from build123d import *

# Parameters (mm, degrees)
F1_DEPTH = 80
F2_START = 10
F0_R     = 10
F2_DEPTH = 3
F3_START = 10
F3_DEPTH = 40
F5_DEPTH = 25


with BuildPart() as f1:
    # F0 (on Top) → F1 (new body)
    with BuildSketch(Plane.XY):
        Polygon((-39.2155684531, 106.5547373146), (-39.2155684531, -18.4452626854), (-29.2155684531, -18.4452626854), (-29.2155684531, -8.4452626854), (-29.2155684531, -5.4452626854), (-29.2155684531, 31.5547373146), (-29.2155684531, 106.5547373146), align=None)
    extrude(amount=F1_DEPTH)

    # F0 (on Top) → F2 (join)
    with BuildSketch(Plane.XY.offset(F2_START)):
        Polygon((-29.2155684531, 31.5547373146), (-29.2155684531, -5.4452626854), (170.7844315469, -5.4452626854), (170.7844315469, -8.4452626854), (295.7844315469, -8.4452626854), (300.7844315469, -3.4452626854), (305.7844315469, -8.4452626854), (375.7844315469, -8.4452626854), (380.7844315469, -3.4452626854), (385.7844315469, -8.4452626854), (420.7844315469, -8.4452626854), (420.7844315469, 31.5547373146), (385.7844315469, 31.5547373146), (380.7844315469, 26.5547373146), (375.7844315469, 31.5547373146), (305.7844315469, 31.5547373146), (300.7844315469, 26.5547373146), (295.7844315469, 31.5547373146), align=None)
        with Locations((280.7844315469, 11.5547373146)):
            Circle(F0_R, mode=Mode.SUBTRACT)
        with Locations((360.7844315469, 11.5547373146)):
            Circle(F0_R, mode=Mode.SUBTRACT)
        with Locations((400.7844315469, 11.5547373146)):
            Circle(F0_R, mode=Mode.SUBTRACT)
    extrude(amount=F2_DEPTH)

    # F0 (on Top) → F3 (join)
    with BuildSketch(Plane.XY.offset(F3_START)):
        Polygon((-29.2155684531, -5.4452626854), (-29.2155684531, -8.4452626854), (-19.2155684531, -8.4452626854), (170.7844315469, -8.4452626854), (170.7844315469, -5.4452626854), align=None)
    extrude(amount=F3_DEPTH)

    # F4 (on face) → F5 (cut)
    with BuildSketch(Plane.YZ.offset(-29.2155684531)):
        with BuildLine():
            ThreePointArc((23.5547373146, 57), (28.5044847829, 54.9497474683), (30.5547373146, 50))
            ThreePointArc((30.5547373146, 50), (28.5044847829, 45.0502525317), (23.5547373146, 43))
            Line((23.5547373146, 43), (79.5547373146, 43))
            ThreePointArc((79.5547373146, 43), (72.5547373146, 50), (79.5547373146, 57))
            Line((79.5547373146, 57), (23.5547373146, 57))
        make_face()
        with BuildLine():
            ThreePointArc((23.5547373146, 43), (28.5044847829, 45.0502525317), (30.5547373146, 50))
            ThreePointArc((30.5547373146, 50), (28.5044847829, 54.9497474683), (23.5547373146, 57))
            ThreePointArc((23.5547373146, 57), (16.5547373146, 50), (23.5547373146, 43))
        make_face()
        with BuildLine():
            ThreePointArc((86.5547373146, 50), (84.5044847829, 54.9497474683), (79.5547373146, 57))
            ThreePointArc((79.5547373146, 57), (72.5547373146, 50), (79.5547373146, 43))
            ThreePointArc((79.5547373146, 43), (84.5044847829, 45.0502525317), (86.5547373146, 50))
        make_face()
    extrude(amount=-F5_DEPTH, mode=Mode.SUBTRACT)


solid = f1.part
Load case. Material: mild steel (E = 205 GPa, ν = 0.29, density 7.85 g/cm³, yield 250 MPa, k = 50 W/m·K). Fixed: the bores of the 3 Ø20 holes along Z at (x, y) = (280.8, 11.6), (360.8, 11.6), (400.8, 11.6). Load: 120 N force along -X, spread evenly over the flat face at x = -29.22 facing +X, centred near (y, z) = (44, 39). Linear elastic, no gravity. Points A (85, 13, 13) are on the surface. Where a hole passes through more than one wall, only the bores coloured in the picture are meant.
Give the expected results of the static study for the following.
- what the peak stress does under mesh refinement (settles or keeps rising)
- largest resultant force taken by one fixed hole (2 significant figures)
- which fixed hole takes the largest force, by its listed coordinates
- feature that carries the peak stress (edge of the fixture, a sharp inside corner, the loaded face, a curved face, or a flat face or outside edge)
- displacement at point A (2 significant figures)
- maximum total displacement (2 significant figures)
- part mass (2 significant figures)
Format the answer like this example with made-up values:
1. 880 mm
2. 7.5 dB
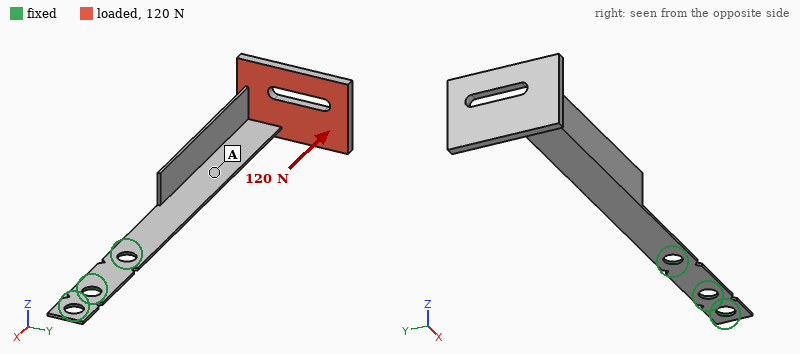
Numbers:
1. keeps rising
2. 120 N
3. (280.8, 11.6)
4. a sharp inside corner
5. 2.6 mm
6. 5.4 mm
7. 1.3 kg
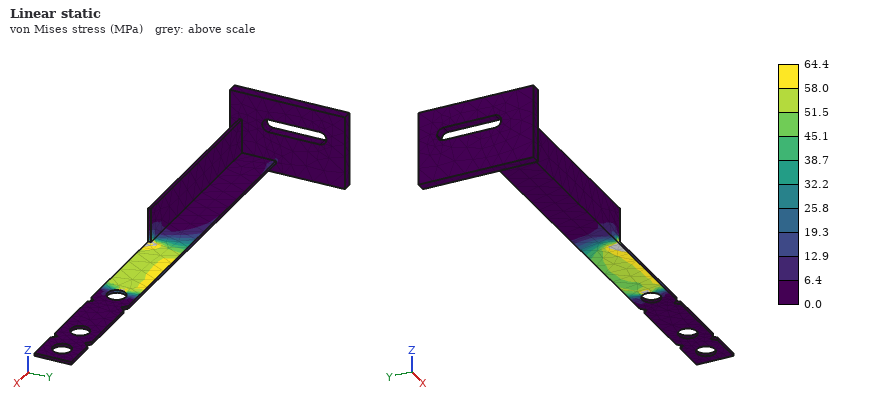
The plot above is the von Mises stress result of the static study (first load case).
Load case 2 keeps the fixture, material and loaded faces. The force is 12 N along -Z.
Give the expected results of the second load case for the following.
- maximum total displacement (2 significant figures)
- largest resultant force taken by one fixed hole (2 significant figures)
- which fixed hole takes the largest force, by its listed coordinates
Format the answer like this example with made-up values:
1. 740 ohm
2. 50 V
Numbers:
1. 5.0 mm
2. 12 N
3. (280.8, 11.6)
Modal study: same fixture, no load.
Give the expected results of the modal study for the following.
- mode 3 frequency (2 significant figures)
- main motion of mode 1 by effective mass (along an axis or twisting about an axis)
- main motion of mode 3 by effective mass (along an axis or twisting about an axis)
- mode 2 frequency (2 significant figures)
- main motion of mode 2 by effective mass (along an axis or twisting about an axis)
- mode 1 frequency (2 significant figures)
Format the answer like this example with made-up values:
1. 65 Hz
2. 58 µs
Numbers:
1. 110 Hz
2. along Z
3. along Y
4. 39 Hz
5. along Y
6. 8.7 Hz
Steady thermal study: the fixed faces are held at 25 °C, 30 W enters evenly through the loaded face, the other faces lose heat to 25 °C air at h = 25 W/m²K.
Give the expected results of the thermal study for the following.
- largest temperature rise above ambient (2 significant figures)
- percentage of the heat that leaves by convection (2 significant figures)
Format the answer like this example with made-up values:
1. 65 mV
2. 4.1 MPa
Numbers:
1. 59 K
2. 100 %
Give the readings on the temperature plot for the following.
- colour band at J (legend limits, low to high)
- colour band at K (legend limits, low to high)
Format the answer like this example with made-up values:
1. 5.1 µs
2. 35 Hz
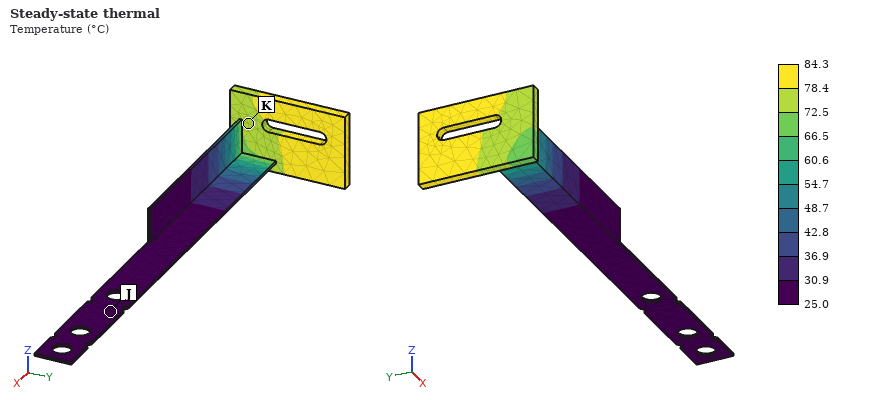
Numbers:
1. 25.0 to 30.9 °C
2. 72.5 to 78.4 °C
